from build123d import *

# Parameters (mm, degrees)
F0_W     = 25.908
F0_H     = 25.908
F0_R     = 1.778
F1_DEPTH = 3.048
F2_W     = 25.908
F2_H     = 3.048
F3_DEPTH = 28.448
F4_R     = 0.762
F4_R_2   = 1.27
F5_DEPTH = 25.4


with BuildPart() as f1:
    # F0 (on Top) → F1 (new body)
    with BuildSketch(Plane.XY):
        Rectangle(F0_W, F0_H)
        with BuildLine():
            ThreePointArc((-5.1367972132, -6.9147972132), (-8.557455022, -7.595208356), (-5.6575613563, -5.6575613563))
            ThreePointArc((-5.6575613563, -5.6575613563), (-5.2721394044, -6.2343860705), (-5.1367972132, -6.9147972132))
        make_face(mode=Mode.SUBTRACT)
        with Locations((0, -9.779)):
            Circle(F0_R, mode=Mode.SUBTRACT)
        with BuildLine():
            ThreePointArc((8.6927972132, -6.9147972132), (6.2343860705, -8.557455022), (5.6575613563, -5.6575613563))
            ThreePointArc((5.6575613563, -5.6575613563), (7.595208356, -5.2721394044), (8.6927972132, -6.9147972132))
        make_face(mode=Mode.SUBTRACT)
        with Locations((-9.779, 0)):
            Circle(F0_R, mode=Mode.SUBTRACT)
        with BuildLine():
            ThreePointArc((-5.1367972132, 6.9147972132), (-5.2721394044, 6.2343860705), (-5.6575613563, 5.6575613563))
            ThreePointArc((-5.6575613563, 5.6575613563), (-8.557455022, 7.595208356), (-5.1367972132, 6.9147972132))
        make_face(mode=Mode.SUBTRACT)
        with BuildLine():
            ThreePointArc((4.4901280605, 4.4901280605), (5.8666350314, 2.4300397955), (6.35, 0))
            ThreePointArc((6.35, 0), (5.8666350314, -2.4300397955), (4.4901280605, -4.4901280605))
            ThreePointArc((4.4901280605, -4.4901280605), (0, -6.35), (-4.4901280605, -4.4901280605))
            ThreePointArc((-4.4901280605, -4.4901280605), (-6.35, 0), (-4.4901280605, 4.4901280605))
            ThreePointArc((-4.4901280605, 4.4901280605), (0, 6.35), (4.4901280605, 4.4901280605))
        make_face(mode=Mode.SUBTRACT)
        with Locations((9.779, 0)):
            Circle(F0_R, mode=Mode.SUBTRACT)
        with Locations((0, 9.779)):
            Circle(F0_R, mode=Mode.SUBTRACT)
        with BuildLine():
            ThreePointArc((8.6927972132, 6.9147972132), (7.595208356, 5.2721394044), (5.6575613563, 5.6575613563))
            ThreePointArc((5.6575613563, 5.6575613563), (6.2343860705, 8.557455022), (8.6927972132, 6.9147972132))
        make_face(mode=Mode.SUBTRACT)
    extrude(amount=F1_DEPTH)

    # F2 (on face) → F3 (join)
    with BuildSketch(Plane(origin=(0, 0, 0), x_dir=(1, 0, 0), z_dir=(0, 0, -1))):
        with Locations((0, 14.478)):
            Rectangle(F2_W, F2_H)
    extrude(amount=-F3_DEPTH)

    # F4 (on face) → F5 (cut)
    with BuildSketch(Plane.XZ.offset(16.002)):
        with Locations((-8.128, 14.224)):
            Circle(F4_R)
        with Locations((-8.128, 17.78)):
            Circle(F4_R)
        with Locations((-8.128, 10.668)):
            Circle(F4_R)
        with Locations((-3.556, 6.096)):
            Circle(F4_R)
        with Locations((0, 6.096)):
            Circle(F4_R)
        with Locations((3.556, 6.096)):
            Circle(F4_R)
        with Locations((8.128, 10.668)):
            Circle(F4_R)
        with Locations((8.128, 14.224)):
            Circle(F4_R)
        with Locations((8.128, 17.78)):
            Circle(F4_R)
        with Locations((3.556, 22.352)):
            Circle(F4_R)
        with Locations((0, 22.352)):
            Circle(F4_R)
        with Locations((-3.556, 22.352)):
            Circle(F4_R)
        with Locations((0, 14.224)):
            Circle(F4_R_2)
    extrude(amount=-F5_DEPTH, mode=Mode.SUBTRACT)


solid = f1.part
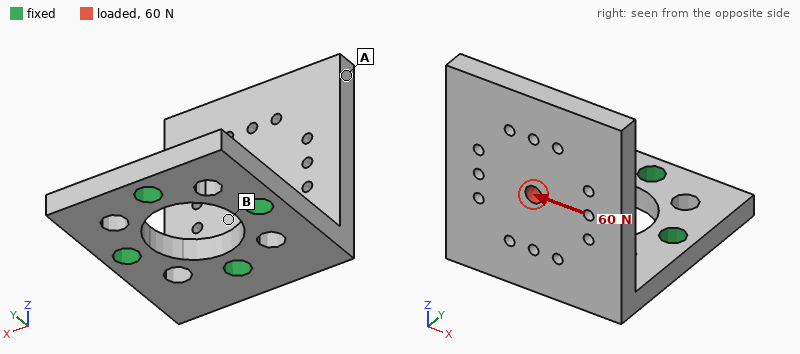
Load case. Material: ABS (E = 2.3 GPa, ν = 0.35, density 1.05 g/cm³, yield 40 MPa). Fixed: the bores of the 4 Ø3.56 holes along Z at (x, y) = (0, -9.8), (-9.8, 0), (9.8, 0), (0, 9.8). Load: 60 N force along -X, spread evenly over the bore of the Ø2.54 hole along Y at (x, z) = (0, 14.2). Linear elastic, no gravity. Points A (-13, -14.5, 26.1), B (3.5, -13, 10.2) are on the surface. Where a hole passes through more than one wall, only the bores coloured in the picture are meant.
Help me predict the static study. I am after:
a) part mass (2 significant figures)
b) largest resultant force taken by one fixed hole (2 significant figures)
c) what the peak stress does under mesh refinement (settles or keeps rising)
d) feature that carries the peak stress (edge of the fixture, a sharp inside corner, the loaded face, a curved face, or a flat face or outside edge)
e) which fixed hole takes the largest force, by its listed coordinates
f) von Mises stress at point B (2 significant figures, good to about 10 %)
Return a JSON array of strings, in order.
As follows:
["3.8 g", "56 N", "keeps rising", "edge of the fixture", "(0, -9.8)", "3.8 MPa"]
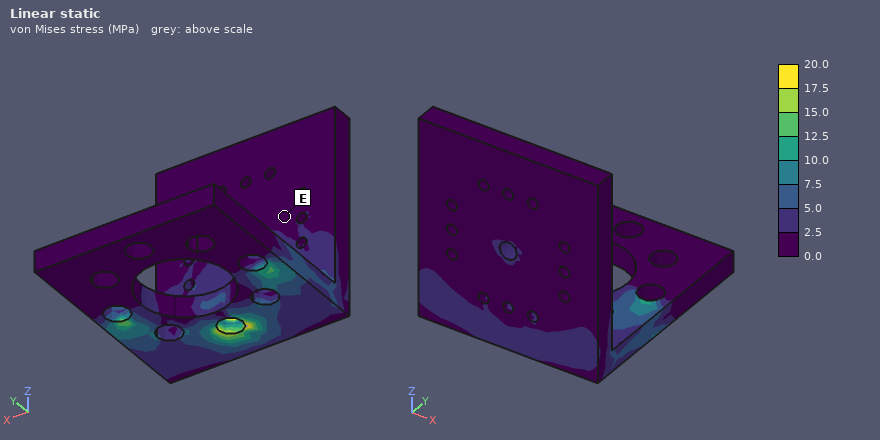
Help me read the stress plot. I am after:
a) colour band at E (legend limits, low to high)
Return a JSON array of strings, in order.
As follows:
["0.0 to 2.5 MPa"]
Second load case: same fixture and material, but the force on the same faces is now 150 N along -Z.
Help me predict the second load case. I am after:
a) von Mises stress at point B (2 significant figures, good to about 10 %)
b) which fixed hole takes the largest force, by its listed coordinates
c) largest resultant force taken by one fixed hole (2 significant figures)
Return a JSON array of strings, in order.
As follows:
["3.3 MPa", "(0, -9.8)", "160 N"]
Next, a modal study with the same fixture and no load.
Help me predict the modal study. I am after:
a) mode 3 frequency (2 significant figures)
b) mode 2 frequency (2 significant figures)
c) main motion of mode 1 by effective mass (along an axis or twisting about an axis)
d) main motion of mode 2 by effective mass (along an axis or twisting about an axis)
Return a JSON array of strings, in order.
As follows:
["2200 Hz", "1400 Hz", "along Y", "along X"]
